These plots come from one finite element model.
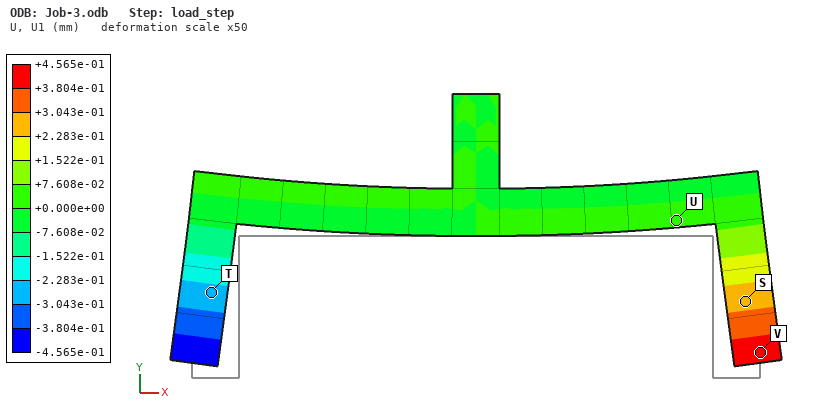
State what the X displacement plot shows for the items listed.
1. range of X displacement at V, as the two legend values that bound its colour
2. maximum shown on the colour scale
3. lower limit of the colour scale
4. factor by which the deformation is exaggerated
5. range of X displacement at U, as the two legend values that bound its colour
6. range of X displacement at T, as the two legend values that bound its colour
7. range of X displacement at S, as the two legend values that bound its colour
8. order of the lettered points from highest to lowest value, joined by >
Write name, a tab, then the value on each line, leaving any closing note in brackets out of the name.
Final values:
range of X displacement at V, as the two legend values that bound its colour	+3.804e-01 to +4.565e-01 mm
maximum shown on the colour scale	+4.565e-01 mm
lower limit of the colour scale	-4.565e-01 mm
factor by which the deformation is exaggerated	50
range of X displacement at U, as the two legend values that bound its colour	+0.000e+00 to +7.608e-02 mm
range of X displacement at T, as the two legend values that bound its colour	-3.043e-01 to -2.283e-01 mm
range of X displacement at S, as the two legend values that bound its colour	+2.283e-01 to +3.043e-01 mm
order of the lettered points from highest to lowest value, joined by >	V > S > U > T
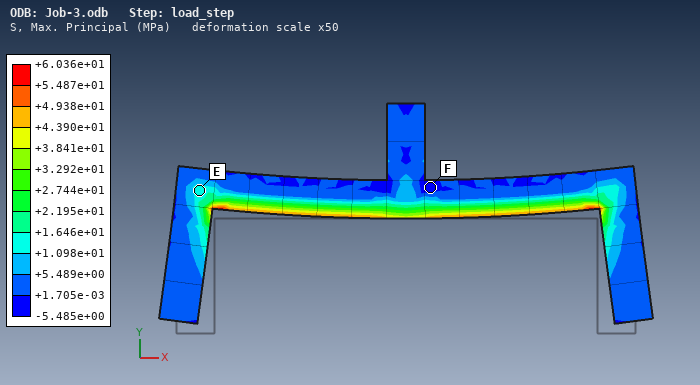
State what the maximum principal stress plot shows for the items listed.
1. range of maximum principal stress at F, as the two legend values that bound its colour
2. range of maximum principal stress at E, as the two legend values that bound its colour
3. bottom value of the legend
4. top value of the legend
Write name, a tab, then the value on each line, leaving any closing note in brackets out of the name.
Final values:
range of maximum principal stress at F, as the two legend values that bound its colour	-5.485e+00 to +1.705e-03 MPa
range of maximum principal stress at E, as the two legend values that bound its colour	+1.098e+01 to +1.646e+01 MPa
bottom value of the legend	-5.485e+00 MPa
top value of the legend	+6.036e+01 MPa
